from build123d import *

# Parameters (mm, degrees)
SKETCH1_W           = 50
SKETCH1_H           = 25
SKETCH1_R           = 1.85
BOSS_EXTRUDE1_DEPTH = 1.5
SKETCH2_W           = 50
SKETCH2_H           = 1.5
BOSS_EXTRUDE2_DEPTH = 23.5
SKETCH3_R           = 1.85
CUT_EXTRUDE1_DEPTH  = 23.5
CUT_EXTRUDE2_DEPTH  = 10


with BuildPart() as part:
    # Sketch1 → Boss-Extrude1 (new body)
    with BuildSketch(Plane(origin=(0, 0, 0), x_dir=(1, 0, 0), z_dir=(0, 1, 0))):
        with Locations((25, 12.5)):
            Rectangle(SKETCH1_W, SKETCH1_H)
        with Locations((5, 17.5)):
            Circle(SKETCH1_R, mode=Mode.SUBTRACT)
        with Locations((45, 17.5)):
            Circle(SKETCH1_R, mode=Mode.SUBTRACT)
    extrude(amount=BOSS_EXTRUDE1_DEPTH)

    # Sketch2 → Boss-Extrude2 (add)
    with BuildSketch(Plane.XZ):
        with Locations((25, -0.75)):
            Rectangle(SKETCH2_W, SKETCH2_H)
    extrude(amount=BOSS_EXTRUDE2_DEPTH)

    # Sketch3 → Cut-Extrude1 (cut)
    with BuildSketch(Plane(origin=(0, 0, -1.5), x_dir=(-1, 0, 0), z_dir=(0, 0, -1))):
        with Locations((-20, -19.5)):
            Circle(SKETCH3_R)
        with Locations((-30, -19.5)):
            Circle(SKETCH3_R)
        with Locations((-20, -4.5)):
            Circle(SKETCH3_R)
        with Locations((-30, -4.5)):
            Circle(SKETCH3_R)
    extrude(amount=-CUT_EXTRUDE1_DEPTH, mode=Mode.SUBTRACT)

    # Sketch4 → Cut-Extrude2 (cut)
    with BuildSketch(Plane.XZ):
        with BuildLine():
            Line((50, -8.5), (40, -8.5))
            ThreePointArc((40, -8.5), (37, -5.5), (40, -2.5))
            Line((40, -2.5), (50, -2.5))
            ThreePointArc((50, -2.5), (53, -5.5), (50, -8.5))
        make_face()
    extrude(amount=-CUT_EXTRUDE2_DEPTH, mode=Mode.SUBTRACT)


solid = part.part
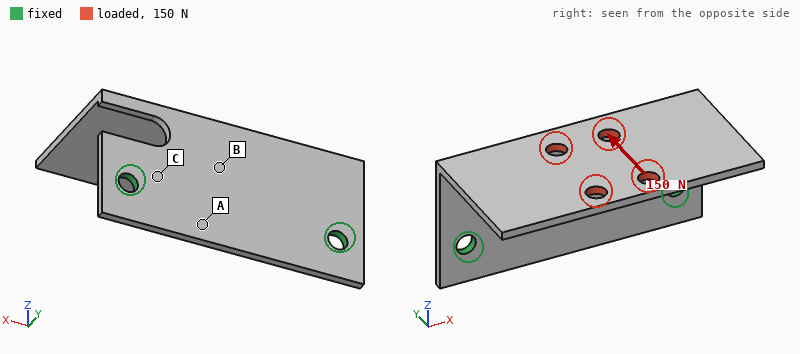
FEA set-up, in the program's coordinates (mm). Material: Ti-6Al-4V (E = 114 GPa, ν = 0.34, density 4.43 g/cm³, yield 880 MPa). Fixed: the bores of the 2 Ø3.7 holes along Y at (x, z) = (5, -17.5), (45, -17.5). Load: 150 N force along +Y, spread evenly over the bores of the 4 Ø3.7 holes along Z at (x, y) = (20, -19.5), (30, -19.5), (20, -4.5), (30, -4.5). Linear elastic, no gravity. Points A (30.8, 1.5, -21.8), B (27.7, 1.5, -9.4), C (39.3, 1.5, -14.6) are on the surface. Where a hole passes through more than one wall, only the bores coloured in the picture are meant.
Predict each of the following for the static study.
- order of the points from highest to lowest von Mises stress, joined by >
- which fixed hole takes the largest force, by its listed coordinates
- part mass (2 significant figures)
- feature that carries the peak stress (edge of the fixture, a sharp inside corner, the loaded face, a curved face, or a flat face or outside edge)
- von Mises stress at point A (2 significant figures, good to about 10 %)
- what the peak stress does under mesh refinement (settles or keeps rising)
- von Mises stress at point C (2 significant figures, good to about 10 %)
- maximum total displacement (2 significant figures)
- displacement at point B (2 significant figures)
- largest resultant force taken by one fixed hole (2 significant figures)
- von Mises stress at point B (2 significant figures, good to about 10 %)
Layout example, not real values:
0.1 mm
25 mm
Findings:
C > B > A
(45, -17.5)
15 g
edge of the fixture
33 MPa
keeps rising
130 MPa
0.65 mm
0.12 mm
80 N
67 MPa
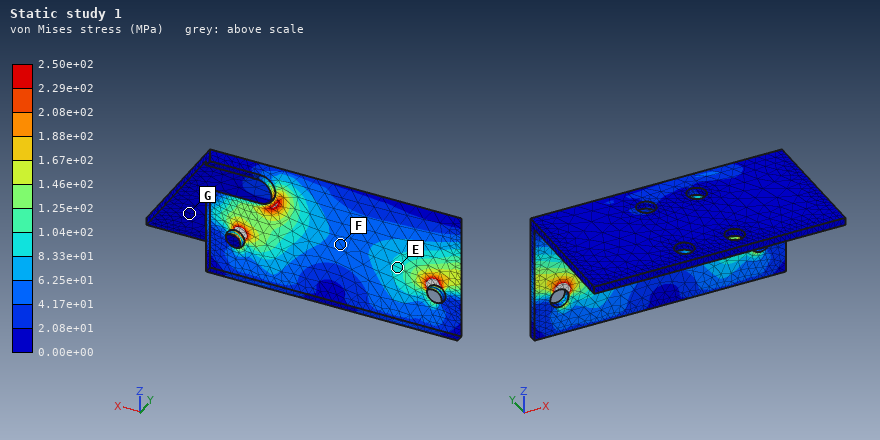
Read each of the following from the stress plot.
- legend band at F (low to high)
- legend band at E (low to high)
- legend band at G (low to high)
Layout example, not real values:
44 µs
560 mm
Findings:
4.17e+01 to 6.25e+01 MPa
8.33e+01 to 1.04e+02 MPa
0.00e+00 to 2.08e+01 MPa
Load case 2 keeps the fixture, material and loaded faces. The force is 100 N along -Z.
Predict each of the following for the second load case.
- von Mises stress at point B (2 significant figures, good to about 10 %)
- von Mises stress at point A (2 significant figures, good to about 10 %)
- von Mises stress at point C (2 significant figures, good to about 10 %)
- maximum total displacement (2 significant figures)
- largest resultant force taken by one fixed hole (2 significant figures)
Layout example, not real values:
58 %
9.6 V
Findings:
68 MPa
25 MPa
65 MPa
0.64 mm
57 N
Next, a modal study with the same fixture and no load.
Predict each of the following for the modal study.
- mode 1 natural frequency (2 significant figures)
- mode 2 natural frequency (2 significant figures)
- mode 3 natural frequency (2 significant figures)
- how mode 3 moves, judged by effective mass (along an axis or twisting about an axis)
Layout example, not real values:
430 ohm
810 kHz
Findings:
810 Hz
1500 Hz
2100 Hz
along Y
